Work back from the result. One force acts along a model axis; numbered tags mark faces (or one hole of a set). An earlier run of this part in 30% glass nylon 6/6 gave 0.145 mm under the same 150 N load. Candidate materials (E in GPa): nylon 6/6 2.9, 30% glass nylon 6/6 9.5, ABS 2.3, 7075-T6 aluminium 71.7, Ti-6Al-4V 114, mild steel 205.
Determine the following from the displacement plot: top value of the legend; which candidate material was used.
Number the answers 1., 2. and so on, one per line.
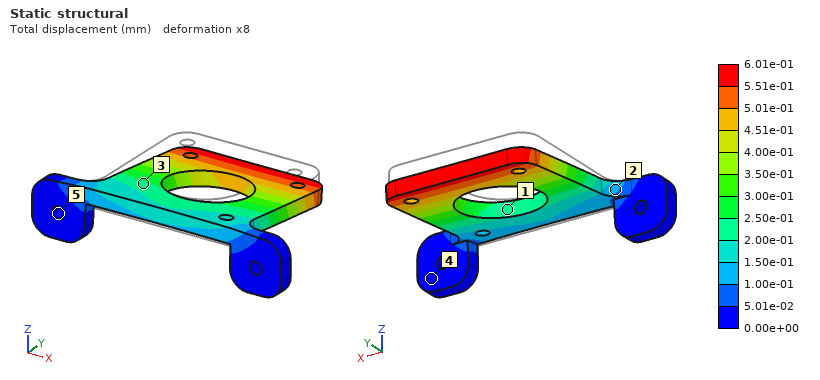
1. 6.01e-01 mm
2. ABS
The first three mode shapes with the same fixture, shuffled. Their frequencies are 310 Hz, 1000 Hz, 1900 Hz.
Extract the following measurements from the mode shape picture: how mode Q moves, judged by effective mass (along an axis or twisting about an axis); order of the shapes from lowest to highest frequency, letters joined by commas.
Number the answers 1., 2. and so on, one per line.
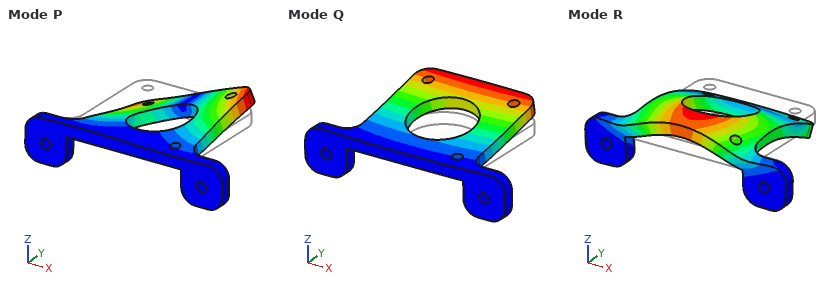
1. along Z
2. Q, P, R
